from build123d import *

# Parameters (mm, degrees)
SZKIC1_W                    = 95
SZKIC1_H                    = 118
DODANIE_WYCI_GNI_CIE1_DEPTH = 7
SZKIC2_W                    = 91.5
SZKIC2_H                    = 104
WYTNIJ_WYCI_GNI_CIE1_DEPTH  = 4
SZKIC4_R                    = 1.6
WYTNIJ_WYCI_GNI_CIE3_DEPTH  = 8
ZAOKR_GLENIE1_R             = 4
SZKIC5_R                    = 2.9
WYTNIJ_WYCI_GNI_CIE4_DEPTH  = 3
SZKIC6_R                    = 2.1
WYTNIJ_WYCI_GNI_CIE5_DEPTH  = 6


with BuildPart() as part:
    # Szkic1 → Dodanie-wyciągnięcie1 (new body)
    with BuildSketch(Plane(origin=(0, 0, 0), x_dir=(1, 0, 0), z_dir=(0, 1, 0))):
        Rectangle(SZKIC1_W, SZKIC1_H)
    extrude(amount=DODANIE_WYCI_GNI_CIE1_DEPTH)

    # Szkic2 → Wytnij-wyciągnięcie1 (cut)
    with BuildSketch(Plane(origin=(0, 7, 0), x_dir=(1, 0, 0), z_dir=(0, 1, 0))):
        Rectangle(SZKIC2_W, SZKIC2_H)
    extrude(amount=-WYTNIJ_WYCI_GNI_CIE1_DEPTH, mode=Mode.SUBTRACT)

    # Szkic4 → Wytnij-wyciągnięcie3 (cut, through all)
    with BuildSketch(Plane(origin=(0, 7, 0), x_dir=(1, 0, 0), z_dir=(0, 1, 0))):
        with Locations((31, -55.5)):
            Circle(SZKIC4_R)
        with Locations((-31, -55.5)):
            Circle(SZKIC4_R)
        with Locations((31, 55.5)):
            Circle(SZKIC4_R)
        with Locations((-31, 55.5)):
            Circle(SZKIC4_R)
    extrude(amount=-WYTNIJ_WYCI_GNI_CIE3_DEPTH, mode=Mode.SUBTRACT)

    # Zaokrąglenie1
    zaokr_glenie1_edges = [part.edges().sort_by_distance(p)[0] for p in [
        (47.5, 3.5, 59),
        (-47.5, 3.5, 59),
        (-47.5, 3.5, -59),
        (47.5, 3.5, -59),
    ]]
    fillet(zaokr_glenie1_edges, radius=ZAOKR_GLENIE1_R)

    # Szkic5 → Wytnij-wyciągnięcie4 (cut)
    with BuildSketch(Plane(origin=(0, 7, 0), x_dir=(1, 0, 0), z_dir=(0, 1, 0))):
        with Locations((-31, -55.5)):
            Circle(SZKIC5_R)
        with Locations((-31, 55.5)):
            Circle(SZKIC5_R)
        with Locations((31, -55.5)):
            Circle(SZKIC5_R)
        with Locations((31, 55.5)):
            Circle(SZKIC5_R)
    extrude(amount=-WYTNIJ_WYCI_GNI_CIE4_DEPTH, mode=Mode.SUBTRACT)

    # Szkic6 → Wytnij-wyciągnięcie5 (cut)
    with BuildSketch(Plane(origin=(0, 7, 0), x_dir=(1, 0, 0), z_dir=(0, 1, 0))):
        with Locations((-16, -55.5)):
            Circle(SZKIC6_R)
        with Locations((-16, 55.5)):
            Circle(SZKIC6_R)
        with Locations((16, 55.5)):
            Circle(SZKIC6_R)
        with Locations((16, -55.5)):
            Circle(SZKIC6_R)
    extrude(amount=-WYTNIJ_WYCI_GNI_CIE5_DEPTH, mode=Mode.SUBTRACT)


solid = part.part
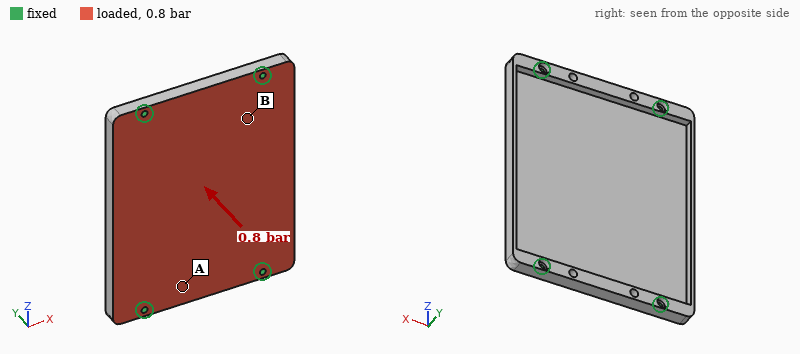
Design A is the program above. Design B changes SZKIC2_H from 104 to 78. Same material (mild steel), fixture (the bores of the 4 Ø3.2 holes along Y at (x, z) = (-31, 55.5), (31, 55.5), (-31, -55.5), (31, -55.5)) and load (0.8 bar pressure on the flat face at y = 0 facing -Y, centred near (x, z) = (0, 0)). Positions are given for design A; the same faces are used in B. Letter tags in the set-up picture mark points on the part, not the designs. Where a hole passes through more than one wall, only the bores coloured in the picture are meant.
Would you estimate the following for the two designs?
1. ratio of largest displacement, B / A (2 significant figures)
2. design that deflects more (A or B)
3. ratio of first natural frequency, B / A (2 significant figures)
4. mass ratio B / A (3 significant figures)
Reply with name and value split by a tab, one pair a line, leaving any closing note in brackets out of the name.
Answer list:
ratio of largest displacement, B / A	0.64
design that deflects more	A
ratio of first natural frequency, B / A	1.2
mass ratio B / A	1.24
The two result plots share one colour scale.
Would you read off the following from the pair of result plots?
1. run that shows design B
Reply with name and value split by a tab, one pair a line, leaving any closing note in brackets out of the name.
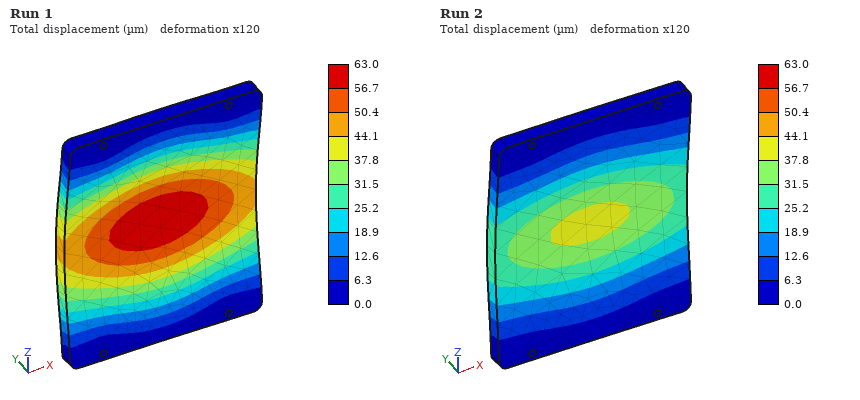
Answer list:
run that shows design B	Run 2
